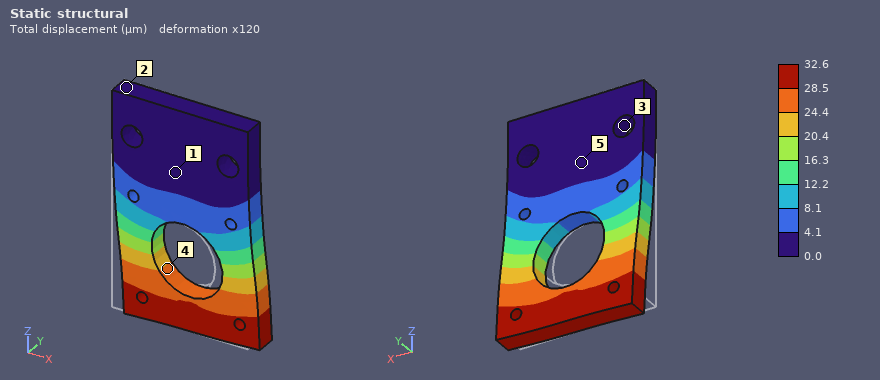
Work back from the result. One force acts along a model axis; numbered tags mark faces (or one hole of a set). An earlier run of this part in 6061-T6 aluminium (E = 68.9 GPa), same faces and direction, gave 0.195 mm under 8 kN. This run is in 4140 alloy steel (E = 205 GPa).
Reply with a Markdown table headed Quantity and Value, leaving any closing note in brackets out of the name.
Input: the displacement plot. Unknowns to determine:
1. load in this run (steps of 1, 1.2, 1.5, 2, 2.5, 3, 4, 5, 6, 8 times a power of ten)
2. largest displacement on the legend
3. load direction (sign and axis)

| Quantity | Value |
|---|---|
| load in this run | 4 kN |
| largest displacement on the legend | 32.6 µm |
| load direction | +X |
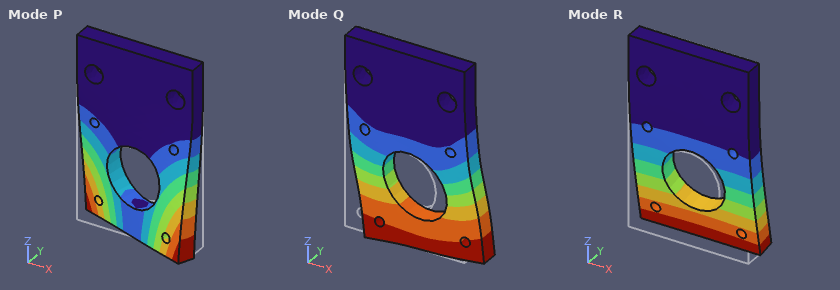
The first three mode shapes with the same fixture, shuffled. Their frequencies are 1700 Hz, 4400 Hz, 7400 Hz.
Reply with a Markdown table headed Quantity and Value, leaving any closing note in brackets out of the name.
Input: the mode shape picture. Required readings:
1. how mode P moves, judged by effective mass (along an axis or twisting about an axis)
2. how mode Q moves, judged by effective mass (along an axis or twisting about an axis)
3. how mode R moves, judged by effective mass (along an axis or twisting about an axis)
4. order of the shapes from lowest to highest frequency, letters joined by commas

| Quantity | Value |
|---|---|
| how mode P moves, judged by effective mass | twisting about Z |
| how mode Q moves, judged by effective mass | along X |
| how mode R moves, judged by effective mass | along Y |
| order of the shapes from lowest to highest frequency, letters joined by commas | R, P, Q |
